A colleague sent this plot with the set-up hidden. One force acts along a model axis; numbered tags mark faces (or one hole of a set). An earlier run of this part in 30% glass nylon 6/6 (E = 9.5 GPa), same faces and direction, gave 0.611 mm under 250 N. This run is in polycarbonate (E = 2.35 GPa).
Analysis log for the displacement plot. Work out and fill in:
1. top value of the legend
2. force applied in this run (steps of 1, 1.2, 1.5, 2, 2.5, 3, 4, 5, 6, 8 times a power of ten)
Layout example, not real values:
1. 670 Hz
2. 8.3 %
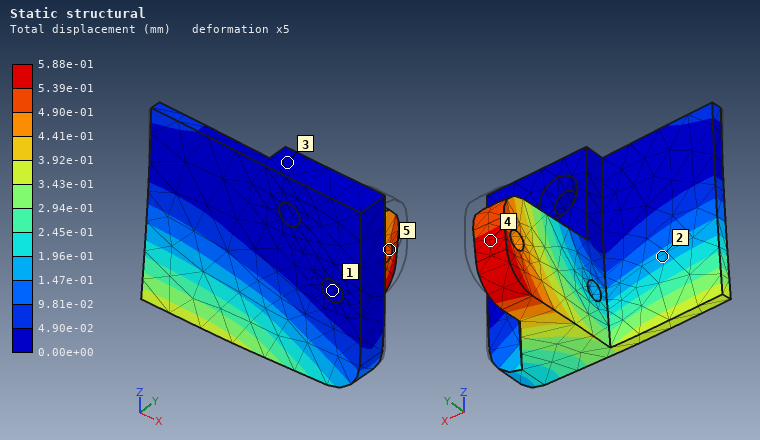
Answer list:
1. 5.88e-01 mm
2. 60 N
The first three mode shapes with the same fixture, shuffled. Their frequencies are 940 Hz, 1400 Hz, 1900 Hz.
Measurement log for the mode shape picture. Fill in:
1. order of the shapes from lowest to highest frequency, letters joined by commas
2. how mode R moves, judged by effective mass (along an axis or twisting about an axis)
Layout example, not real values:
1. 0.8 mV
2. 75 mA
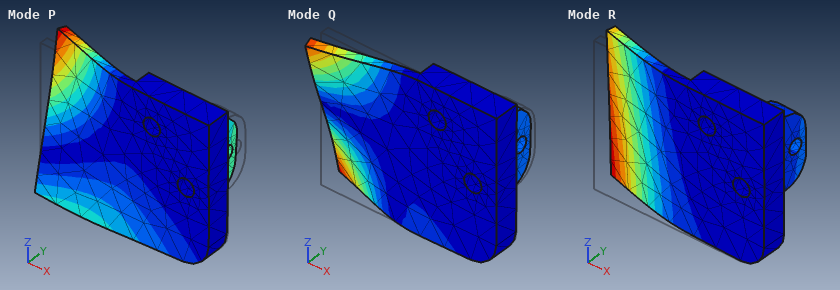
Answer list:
1. R, P, Q
2. along Y
